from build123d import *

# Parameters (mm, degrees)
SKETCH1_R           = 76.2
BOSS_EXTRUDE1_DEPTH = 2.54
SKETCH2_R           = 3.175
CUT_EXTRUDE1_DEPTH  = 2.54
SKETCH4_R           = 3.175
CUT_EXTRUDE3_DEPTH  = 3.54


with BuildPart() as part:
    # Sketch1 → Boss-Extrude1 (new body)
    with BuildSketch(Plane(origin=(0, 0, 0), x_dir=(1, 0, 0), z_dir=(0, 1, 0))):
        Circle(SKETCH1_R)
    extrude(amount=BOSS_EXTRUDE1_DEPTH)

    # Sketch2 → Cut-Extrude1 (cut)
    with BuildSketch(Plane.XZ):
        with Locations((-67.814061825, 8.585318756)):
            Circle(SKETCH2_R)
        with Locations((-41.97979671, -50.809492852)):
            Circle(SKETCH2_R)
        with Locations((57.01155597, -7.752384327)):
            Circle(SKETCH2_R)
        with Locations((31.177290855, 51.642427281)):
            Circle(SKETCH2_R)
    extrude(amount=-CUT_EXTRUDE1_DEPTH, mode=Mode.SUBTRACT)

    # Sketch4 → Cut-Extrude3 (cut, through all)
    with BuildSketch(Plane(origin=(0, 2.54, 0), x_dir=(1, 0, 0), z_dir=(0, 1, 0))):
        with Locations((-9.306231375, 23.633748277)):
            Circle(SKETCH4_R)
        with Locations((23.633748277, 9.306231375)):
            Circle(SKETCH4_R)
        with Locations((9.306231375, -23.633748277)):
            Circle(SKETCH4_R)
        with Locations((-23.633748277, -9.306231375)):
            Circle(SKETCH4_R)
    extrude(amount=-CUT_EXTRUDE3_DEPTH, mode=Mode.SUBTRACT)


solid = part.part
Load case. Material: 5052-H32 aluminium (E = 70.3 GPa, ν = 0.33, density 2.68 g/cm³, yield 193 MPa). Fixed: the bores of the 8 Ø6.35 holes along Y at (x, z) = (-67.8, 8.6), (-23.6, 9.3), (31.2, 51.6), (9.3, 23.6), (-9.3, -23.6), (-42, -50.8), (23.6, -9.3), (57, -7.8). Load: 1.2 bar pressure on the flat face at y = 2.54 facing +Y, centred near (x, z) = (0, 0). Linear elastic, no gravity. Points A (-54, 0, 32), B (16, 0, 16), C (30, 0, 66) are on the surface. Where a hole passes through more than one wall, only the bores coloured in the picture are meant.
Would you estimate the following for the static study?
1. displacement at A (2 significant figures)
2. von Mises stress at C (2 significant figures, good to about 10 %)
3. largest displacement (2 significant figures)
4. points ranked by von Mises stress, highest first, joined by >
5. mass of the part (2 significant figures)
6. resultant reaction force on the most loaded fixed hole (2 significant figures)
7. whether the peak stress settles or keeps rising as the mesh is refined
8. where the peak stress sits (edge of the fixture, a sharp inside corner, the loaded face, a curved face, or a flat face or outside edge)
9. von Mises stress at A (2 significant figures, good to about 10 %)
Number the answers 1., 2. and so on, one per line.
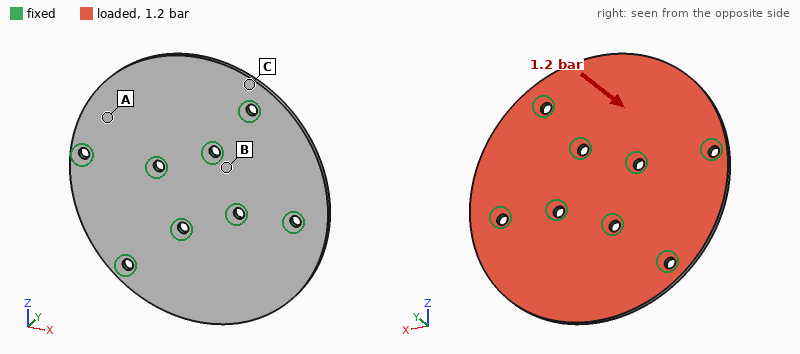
1. 0.22 mm
2. 63 MPa
3. 0.87 mm
4. C > A > B
5. 120 g
6. 330 N
7. keeps rising
8. edge of the fixture
9. 33 MPa
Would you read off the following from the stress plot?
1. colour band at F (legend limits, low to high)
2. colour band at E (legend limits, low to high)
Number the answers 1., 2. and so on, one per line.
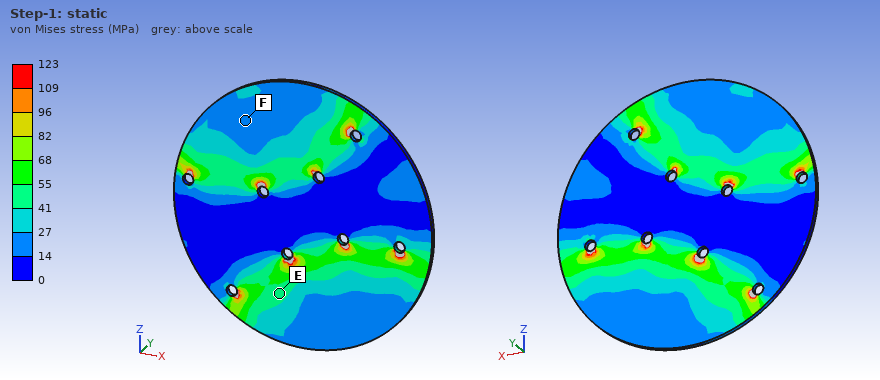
1. 14 to 27 MPa
2. 41 to 55 MPa
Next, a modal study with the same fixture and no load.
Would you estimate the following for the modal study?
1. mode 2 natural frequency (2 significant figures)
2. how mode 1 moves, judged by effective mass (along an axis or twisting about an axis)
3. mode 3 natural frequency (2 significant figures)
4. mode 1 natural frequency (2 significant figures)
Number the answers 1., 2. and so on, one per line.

1. 1000 Hz
2. along Y
3. 2100 Hz
4. 960 Hz
